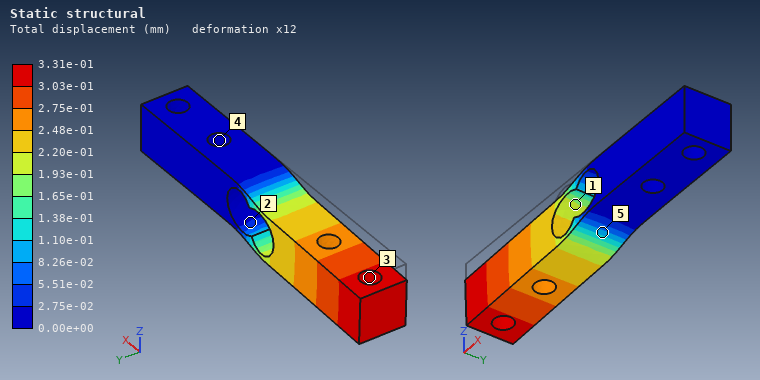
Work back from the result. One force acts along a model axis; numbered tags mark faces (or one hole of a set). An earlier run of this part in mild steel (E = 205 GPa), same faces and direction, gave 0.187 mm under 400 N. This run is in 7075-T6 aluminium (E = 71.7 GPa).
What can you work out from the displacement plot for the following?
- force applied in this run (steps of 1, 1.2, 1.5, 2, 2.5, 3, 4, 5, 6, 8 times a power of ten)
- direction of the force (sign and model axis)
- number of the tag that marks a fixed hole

250 N
-Z
4
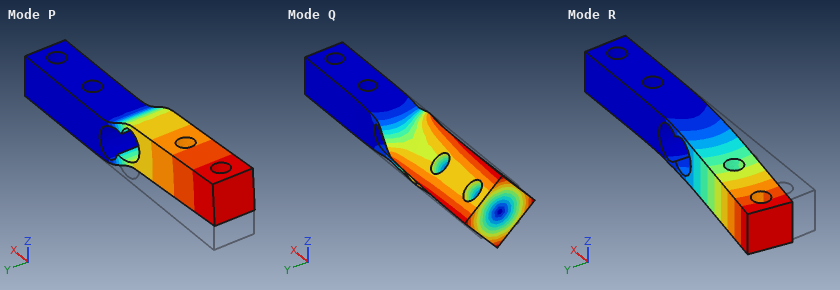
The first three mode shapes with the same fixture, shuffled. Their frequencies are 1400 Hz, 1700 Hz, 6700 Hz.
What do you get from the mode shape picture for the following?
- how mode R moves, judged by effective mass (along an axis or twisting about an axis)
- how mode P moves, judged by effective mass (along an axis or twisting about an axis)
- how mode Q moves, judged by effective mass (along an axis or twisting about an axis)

along Y
along Z
twisting about X
